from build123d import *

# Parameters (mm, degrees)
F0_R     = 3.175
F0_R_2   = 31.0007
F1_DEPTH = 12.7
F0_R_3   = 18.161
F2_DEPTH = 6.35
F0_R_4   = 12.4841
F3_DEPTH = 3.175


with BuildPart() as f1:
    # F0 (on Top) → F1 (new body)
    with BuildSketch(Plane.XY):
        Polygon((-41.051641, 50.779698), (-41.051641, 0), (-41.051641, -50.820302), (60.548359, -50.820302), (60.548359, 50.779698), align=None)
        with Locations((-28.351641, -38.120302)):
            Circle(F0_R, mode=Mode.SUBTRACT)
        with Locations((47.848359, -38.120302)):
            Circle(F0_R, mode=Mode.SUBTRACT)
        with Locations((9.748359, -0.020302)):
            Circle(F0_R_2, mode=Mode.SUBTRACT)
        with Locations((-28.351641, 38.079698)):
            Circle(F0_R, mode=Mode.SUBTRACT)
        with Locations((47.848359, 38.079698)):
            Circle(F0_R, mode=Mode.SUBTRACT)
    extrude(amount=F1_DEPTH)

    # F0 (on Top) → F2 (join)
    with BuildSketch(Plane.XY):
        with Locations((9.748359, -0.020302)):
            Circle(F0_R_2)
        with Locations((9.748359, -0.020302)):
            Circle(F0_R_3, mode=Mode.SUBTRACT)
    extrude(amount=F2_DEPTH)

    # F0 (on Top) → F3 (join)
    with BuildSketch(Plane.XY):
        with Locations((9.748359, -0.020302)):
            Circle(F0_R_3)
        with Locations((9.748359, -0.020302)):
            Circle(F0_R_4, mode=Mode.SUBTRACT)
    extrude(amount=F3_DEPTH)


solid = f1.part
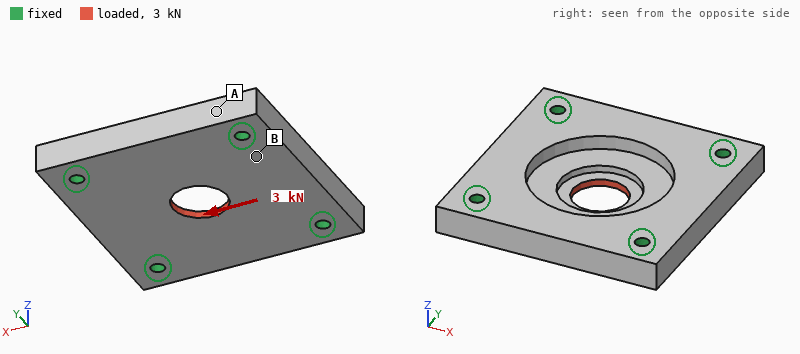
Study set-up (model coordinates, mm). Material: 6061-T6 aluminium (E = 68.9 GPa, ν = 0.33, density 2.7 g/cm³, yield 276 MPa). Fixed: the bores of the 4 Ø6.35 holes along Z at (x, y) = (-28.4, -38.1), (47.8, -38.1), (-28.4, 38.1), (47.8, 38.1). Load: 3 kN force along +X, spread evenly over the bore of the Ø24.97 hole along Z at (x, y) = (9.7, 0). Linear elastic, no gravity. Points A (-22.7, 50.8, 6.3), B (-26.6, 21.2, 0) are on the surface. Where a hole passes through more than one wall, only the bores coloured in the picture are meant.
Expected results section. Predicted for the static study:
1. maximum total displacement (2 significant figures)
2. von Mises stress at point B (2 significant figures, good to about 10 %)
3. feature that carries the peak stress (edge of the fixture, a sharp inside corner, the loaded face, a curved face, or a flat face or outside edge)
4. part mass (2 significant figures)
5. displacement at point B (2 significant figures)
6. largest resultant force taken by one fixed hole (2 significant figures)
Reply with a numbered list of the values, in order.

1. 7.0 µm
2. 3.8 MPa
3. a sharp inside corner
4. 280 g
5. 1.5 µm
6. 820 N
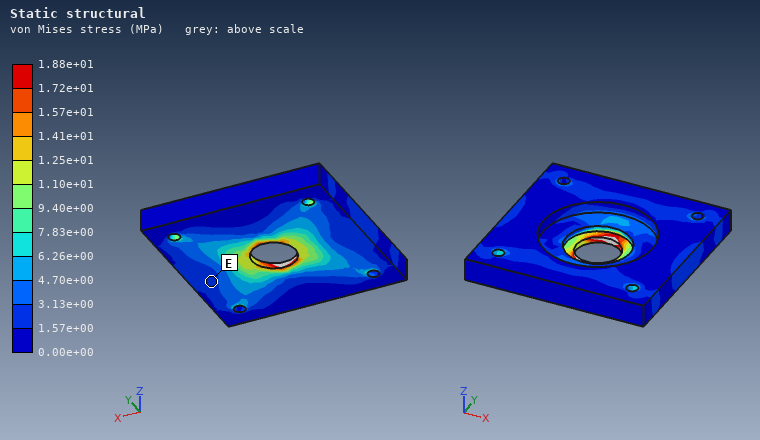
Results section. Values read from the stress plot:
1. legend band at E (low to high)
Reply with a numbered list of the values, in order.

1. 1.57e+00 to 3.13e+00 MPa
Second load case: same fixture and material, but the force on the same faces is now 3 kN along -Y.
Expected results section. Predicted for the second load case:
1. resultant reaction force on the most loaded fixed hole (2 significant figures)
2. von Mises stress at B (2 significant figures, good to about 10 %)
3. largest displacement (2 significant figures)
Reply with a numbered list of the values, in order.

1. 820 N
2. 2.3 MPa
3. 7.0 µm
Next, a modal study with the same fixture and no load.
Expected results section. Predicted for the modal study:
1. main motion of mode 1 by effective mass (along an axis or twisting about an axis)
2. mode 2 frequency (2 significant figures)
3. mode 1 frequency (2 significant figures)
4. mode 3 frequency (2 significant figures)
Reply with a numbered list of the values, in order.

1. along Z
2. 9600 Hz
3. 7800 Hz
4. 9600 Hz
